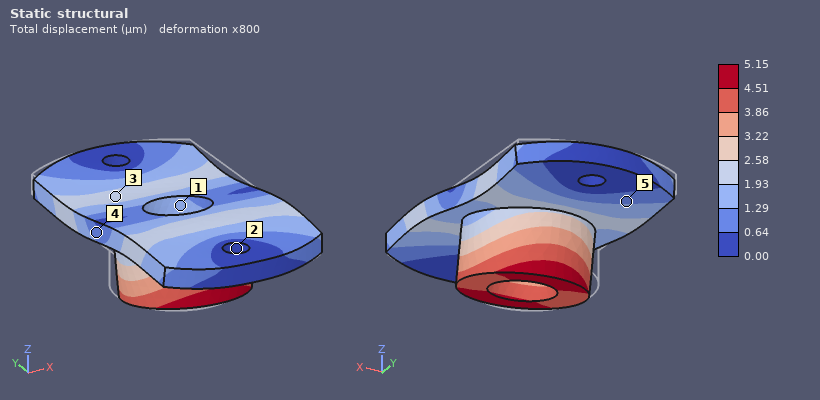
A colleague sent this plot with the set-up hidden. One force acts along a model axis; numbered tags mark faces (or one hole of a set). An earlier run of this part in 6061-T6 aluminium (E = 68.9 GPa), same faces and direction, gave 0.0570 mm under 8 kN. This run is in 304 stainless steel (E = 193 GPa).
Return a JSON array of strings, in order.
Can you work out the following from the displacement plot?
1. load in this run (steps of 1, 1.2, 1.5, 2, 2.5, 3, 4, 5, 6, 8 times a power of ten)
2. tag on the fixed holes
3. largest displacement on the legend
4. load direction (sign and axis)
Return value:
["2 kN", "2", "5.15 µm", "-Y"]
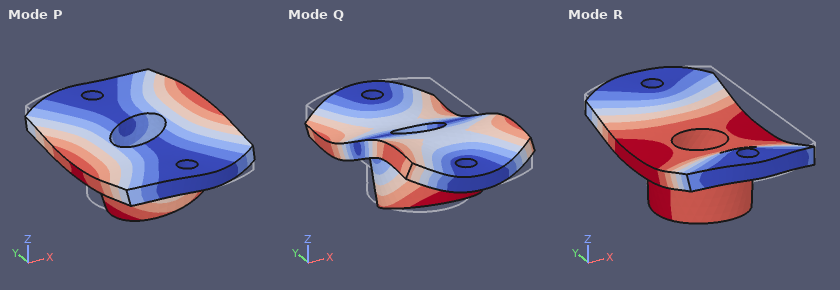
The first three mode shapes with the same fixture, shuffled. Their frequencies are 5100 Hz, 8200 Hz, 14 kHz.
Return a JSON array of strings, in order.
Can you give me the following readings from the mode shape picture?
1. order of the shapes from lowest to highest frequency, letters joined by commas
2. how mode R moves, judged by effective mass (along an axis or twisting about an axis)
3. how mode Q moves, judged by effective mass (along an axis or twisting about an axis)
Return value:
["P, R, Q", "along Z", "along Y"]
